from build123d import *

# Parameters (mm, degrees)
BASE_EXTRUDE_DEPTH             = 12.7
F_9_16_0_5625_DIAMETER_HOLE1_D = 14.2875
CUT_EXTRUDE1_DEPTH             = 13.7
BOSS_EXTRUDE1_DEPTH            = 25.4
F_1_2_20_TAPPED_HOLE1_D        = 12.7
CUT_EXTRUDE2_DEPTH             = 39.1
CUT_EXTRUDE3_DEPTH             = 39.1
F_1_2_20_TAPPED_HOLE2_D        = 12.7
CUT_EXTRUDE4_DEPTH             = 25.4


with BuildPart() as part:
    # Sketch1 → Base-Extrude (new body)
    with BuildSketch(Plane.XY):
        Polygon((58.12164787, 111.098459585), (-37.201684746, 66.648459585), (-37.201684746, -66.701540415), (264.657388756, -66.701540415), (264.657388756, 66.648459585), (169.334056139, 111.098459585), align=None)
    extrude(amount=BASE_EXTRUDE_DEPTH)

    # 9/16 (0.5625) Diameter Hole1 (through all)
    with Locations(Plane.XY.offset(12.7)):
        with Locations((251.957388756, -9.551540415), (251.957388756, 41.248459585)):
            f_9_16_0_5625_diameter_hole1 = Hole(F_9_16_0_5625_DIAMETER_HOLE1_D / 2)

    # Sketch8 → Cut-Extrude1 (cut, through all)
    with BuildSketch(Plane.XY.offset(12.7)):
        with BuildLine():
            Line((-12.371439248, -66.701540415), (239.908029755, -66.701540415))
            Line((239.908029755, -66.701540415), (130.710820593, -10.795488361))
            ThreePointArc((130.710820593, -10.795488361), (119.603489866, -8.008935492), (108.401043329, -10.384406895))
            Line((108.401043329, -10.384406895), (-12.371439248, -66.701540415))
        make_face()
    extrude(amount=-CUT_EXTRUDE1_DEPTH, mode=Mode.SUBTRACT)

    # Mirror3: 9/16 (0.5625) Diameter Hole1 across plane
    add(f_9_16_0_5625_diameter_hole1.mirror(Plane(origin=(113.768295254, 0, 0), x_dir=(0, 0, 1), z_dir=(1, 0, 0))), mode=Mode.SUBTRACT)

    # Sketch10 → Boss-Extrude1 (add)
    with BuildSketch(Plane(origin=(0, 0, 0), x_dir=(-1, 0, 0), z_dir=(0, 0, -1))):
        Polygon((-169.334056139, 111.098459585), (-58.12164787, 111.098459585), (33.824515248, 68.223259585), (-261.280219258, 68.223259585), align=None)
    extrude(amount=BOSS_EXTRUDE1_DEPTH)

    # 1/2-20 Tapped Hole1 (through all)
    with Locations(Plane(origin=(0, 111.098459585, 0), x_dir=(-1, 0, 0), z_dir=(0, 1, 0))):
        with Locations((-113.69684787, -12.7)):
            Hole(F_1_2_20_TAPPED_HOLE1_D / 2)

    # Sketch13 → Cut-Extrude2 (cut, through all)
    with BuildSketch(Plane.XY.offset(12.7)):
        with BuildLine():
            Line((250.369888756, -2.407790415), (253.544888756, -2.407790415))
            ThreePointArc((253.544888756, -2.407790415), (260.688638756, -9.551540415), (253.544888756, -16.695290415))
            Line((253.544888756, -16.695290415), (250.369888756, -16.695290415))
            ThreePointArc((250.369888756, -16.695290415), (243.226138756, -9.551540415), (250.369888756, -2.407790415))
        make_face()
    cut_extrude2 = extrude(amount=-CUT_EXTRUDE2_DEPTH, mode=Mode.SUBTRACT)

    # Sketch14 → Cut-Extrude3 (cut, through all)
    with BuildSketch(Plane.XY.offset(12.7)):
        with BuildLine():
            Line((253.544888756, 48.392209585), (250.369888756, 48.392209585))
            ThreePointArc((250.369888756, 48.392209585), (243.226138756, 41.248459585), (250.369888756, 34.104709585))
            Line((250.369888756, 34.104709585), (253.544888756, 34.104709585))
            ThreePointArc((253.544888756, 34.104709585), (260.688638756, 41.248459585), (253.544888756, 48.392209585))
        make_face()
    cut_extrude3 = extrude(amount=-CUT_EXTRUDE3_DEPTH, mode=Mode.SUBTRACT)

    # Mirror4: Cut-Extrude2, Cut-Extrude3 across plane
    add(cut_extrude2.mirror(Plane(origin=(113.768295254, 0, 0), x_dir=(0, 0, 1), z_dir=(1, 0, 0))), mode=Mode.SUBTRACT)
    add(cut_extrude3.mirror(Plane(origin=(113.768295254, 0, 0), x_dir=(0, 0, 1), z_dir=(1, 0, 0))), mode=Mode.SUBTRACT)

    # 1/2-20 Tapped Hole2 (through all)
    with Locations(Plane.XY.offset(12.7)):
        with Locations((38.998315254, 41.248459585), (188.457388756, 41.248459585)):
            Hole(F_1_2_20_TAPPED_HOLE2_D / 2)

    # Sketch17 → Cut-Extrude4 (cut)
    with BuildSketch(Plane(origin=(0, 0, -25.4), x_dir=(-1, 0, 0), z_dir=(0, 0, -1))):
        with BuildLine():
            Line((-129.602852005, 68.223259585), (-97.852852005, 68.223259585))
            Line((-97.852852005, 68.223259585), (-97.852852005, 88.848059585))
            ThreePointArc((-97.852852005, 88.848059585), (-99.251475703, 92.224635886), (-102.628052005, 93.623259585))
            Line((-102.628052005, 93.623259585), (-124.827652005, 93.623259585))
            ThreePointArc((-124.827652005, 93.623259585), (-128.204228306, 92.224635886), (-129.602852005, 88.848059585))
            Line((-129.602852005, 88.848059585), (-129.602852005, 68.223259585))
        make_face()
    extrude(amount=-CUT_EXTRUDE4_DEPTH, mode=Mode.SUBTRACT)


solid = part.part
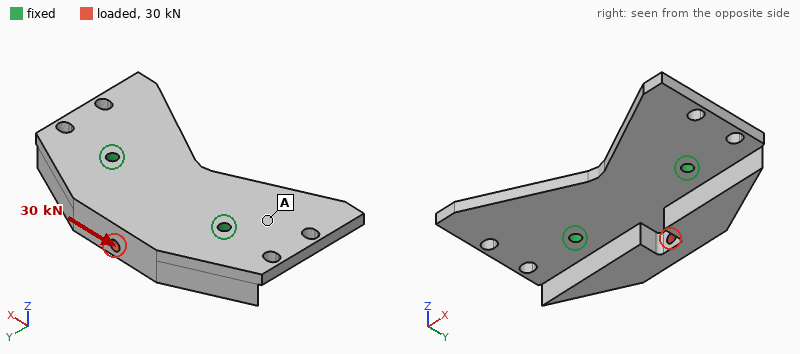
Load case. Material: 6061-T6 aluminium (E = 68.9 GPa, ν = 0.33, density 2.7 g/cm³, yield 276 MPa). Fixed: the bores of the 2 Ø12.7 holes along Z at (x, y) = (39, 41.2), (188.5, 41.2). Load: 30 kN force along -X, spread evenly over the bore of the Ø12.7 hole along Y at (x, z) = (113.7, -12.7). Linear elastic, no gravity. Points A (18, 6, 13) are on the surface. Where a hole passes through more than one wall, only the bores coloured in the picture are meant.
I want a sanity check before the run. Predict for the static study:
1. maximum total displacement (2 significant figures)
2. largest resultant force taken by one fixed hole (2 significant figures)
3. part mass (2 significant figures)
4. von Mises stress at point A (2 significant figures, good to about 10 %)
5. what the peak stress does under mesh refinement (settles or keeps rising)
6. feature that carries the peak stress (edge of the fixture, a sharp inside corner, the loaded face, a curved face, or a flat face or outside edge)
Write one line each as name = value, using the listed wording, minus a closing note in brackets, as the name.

maximum total displacement = 78 µm
largest resultant force taken by one fixed hole = 19 kN
part mass = 1.9 kg
von Mises stress at point A = 9.9 MPa
what the peak stress does under mesh refinement = keeps rising
feature that carries the peak stress = edge of the fixture
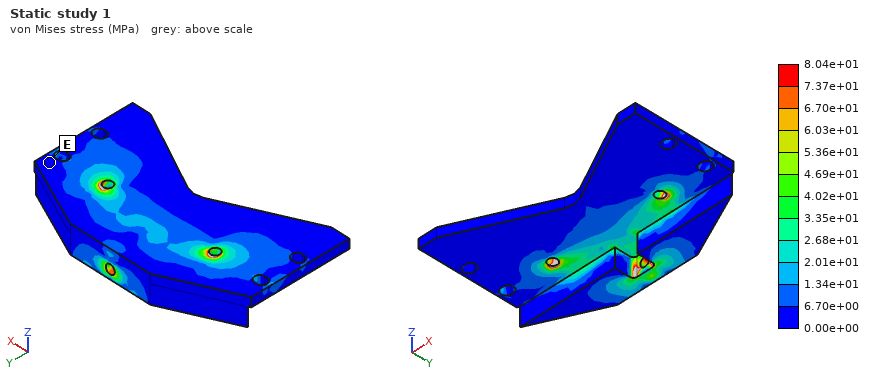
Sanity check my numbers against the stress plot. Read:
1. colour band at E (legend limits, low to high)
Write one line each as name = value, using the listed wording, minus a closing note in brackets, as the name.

colour band at E = 0.00e+00 to 6.70e+00 MPa
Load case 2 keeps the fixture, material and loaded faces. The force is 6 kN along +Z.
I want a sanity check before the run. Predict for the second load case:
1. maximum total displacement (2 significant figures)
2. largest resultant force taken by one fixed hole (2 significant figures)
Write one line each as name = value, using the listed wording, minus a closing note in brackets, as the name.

maximum total displacement = 0.33 mm
largest resultant force taken by one fixed hole = 3.1 kN
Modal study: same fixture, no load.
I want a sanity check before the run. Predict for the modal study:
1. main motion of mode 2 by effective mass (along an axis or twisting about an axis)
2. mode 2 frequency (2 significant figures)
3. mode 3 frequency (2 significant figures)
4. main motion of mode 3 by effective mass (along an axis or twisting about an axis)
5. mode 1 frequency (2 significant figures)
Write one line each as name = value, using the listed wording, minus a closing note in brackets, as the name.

main motion of mode 2 by effective mass = twisting about Y
mode 2 frequency = 950 Hz
mode 3 frequency = 1300 Hz
main motion of mode 3 by effective mass = along Z
mode 1 frequency = 850 Hz
